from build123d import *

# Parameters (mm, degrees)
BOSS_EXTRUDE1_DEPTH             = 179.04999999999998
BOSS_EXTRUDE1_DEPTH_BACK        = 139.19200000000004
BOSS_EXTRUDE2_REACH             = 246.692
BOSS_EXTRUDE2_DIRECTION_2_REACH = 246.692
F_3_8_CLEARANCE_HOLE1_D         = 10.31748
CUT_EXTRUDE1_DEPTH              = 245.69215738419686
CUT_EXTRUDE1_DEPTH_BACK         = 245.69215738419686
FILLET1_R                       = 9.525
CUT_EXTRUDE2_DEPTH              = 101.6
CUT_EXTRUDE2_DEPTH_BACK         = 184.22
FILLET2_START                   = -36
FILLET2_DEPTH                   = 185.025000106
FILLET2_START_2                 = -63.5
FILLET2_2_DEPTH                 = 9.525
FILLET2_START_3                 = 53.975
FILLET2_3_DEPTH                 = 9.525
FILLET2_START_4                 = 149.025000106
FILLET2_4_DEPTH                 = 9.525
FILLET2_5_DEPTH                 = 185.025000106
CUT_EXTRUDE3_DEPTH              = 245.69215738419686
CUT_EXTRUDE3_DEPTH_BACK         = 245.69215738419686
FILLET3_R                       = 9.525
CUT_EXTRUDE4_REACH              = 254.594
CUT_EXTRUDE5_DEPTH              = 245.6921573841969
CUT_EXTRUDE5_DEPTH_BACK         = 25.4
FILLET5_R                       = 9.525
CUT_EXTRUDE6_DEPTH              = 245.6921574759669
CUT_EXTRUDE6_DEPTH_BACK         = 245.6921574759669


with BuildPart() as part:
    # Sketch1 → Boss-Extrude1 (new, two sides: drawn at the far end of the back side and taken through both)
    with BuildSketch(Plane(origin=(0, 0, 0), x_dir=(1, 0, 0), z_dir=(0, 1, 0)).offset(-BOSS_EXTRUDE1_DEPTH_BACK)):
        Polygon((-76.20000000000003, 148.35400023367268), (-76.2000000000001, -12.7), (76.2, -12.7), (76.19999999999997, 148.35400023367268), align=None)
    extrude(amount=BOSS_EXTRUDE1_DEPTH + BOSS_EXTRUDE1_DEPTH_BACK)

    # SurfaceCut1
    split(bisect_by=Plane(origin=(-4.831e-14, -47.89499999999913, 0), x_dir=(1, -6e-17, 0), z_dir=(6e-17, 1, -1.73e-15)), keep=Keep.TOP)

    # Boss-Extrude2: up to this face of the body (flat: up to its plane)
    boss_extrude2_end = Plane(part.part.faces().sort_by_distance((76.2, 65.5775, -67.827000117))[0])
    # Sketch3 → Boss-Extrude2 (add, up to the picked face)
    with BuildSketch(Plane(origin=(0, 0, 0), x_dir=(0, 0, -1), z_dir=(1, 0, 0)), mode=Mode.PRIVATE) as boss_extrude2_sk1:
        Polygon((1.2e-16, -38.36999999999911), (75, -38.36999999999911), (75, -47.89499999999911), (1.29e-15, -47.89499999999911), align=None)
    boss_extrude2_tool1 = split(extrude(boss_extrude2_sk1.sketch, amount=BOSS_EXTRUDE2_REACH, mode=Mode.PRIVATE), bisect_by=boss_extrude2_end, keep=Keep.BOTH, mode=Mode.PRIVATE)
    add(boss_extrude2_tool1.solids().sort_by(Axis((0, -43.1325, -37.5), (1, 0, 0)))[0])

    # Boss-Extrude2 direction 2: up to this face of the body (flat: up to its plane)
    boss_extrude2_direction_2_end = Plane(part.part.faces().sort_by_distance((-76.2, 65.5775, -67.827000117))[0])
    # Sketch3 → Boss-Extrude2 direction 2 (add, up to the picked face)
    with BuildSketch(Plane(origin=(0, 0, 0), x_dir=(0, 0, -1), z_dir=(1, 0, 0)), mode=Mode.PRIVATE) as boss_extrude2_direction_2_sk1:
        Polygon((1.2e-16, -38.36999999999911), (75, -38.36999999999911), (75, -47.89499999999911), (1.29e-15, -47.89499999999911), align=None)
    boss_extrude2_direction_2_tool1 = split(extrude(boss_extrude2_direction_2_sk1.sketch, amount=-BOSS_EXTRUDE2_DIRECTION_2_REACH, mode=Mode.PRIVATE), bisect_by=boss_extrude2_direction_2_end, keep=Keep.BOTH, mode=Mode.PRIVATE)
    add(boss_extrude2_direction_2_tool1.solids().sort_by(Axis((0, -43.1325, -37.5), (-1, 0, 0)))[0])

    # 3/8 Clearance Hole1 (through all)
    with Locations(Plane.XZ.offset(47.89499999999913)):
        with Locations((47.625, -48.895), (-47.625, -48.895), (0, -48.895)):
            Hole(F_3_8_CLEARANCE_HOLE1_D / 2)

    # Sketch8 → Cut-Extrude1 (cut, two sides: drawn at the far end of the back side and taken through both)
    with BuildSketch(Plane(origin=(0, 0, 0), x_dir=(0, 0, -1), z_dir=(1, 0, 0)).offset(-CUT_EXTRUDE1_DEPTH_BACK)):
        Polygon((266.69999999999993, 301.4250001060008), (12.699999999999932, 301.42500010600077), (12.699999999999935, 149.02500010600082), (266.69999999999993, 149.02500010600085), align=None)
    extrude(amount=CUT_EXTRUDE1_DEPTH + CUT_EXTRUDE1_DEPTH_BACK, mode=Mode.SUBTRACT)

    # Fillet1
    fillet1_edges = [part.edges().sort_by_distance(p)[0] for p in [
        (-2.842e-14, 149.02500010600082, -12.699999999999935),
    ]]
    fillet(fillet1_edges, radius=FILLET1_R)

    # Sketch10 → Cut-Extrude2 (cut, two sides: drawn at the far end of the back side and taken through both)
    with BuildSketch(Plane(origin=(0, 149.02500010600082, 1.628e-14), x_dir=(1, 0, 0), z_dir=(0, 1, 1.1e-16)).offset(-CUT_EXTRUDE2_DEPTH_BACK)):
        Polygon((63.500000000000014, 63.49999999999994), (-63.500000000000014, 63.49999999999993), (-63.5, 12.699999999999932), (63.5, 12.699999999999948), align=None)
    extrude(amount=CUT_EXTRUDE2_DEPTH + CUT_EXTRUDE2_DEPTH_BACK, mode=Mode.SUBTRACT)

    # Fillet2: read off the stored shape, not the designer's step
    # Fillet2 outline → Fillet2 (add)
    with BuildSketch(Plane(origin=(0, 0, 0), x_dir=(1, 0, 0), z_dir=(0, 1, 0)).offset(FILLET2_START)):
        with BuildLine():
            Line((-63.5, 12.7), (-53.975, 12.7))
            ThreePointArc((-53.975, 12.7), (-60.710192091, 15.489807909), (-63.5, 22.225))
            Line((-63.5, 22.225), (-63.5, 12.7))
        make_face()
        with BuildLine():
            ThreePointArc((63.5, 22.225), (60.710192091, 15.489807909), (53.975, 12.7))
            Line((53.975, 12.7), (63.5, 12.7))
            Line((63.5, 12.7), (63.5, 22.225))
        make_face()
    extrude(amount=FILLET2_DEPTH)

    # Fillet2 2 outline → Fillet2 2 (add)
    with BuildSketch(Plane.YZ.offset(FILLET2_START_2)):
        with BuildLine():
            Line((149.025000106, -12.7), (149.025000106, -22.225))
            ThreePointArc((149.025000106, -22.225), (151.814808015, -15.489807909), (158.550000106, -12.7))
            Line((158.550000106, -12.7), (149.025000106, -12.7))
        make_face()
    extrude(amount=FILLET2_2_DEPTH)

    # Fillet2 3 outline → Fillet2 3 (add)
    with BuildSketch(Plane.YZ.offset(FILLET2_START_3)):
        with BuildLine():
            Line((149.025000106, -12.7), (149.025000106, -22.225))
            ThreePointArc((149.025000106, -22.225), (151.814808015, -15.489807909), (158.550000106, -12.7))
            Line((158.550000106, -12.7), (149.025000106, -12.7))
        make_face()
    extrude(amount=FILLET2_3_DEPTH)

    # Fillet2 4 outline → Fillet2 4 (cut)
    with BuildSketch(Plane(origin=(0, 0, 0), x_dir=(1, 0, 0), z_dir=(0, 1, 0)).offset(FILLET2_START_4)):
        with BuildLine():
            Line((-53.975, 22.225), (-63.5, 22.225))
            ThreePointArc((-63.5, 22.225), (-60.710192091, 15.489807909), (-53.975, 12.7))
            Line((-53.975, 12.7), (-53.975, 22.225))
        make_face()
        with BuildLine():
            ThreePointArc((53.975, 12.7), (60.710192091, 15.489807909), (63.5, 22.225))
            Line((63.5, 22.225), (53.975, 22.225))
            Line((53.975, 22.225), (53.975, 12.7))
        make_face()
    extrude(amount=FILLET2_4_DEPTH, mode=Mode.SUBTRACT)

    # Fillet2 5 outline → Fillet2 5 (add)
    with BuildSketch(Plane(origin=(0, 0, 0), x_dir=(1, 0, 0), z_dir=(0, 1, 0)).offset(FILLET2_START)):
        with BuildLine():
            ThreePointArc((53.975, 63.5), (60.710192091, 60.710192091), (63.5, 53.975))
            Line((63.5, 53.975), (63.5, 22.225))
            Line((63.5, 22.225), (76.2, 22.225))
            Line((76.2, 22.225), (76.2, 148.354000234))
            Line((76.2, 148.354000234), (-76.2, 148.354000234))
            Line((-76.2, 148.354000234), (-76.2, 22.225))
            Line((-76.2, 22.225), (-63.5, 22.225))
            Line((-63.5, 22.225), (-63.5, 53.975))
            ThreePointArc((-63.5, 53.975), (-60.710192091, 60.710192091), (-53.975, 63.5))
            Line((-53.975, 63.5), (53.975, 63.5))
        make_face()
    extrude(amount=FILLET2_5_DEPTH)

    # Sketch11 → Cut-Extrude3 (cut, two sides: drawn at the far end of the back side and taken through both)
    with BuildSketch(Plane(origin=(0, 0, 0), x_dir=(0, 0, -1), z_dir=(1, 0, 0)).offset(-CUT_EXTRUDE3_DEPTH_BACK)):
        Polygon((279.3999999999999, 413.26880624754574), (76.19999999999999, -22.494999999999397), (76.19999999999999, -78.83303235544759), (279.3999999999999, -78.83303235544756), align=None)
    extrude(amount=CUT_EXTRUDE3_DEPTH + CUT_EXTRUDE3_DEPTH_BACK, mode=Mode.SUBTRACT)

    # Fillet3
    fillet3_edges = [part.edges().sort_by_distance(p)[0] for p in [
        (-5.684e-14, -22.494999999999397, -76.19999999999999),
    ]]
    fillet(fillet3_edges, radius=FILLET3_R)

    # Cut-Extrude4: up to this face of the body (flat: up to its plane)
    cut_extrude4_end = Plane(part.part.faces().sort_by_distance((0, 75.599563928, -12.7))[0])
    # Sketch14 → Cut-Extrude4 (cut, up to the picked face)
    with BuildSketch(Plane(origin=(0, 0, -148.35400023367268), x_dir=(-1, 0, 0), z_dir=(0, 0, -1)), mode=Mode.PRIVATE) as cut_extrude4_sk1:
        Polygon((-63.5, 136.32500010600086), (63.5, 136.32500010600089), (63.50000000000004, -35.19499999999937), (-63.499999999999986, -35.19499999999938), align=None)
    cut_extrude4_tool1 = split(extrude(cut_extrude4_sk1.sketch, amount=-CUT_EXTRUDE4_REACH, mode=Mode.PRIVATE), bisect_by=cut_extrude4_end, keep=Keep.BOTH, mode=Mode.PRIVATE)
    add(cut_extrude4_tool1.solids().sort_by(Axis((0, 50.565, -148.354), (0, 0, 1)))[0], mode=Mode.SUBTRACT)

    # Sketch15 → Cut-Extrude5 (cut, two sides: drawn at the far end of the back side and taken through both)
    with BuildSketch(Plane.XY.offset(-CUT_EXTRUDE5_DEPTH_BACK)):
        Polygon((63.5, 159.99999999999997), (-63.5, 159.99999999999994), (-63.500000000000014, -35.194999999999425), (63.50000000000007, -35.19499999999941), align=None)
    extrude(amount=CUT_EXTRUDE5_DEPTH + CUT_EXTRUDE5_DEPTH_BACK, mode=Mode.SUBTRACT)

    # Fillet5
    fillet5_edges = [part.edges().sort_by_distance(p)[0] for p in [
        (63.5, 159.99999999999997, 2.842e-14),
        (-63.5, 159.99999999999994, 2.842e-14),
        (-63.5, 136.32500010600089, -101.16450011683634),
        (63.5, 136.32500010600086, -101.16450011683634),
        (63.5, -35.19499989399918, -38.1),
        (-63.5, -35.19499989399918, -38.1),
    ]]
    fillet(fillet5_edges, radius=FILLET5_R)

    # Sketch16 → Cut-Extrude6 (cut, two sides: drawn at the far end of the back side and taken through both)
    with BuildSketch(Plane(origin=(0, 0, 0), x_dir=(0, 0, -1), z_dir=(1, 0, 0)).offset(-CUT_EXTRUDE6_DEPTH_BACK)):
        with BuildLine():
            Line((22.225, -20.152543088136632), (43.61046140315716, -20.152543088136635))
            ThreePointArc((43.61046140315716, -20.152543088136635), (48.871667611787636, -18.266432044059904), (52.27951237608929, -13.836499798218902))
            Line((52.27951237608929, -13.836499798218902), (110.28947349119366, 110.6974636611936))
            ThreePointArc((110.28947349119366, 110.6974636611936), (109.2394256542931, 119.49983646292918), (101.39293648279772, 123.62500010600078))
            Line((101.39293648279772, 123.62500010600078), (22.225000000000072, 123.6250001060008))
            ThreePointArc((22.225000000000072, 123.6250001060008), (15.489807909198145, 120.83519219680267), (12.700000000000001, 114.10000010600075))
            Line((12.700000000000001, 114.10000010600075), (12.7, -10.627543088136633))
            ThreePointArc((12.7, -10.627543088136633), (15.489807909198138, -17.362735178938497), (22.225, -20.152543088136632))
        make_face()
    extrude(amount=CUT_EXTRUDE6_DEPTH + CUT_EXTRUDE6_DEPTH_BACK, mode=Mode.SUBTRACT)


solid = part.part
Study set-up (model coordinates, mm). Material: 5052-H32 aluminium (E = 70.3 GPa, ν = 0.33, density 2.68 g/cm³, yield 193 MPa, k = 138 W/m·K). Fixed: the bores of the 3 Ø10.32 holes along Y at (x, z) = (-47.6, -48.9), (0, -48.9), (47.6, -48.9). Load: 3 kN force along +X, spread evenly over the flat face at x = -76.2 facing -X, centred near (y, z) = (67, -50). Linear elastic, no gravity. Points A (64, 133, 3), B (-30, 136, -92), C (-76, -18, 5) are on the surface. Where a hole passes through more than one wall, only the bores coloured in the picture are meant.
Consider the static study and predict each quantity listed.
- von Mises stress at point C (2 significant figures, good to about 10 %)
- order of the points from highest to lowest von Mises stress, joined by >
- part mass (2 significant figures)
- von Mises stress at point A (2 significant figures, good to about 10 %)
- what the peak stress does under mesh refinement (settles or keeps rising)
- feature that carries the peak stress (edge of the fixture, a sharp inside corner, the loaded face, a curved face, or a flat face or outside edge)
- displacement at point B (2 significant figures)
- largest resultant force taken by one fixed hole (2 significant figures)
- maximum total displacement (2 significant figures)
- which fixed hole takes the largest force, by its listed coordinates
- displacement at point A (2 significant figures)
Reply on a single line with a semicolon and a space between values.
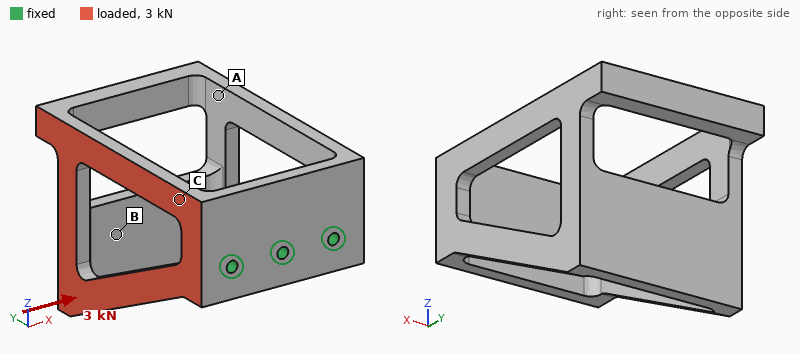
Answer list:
45 MPa; C > A > B; 2.0 kg; 32 MPa; keeps rising; edge of the fixture; 0.97 mm; 2.6 kN; 1.0 mm; (-47.6, -48.9); 0.91 mm
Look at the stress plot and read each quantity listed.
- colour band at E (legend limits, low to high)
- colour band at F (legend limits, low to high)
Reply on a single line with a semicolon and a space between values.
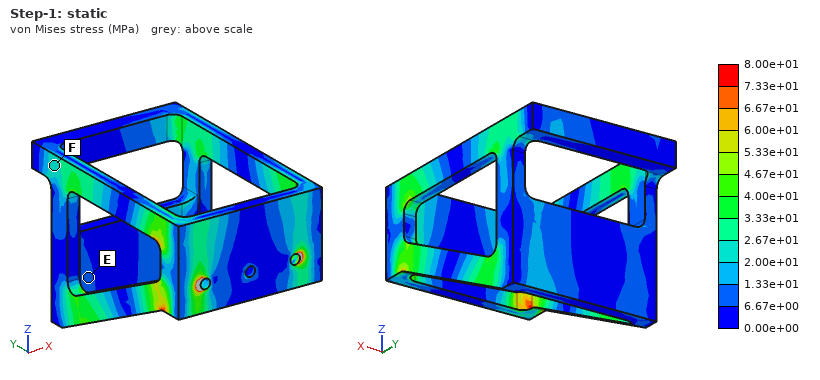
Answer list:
6.67e+00 to 1.33e+01 MPa; 2.00e+01 to 2.67e+01 MPa
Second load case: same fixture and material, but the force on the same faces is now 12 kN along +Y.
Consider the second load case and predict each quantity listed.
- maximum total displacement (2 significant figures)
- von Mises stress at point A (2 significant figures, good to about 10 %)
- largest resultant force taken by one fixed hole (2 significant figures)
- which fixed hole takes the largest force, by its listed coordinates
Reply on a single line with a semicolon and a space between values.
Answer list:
0.74 mm; 14 MPa; 14 kN; (-47.6, -48.9)
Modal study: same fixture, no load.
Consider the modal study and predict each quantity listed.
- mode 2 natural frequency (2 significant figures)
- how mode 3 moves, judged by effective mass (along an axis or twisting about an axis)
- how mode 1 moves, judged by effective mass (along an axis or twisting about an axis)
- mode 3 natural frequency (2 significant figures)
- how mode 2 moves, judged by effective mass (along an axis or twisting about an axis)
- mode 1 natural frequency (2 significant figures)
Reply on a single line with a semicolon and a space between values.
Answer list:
220 Hz; twisting about Y; along X; 390 Hz; along Z; 210 Hz
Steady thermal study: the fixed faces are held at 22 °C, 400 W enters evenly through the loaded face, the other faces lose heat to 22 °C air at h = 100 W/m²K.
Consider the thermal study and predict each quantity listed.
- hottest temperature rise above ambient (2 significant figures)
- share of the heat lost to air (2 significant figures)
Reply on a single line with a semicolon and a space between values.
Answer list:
76 K; 71 %
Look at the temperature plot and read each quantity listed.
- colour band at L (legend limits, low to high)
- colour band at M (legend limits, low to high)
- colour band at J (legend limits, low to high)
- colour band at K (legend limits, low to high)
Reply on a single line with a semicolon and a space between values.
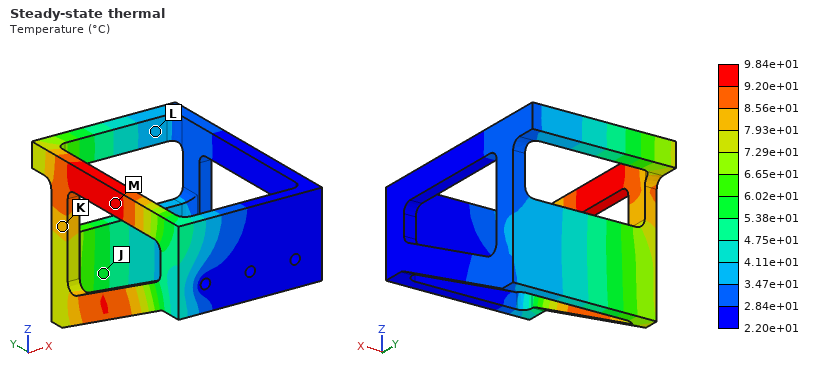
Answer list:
3.47e+01 to 4.11e+01 °C; 9.20e+01 to 9.84e+01 °C; 5.38e+01 to 6.02e+01 °C; 7.93e+01 to 8.56e+01 °C
